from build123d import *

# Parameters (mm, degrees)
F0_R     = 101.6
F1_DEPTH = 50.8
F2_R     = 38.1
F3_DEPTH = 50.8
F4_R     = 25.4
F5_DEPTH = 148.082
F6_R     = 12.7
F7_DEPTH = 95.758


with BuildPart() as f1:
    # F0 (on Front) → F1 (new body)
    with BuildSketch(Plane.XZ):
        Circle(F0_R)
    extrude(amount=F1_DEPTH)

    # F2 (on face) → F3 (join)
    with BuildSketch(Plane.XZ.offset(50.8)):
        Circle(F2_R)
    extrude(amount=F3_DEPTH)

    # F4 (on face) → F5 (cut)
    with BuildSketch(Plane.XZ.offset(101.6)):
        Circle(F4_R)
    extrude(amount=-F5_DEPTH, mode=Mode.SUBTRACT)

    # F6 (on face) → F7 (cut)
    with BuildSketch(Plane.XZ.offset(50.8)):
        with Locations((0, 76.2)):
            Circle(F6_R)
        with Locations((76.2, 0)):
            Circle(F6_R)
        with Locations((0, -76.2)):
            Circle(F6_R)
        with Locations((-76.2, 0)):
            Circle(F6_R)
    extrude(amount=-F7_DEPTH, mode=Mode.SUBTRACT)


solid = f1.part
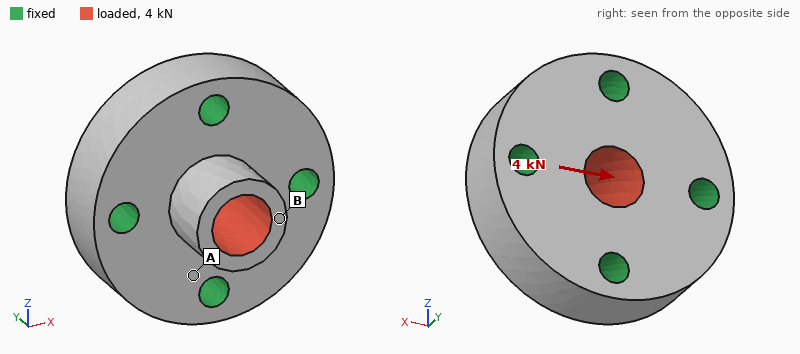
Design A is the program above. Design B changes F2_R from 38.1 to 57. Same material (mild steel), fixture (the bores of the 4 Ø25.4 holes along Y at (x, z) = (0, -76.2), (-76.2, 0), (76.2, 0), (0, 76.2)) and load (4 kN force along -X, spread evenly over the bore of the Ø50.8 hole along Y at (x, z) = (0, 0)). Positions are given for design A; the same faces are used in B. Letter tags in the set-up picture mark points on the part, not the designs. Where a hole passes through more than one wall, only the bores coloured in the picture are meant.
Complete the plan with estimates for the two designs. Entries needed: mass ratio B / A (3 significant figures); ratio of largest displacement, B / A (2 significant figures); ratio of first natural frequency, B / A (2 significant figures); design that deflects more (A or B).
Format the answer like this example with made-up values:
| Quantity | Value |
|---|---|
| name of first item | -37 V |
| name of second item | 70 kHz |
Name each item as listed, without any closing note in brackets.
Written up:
| Quantity | Value |
|---|---|
| mass ratio B / A | 1.18 |
| ratio of largest displacement, B / A | 0.32 |
| ratio of first natural frequency, B / A | 1.0 |
| design that deflects more | A |
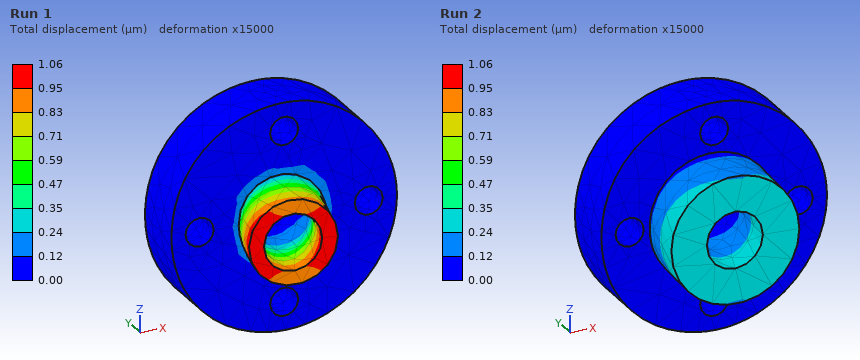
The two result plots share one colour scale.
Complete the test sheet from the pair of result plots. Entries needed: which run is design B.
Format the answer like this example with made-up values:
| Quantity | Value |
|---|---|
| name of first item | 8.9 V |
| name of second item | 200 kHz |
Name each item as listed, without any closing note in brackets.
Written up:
| Quantity | Value |
|---|---|
| which run is design B | Run 2 |
